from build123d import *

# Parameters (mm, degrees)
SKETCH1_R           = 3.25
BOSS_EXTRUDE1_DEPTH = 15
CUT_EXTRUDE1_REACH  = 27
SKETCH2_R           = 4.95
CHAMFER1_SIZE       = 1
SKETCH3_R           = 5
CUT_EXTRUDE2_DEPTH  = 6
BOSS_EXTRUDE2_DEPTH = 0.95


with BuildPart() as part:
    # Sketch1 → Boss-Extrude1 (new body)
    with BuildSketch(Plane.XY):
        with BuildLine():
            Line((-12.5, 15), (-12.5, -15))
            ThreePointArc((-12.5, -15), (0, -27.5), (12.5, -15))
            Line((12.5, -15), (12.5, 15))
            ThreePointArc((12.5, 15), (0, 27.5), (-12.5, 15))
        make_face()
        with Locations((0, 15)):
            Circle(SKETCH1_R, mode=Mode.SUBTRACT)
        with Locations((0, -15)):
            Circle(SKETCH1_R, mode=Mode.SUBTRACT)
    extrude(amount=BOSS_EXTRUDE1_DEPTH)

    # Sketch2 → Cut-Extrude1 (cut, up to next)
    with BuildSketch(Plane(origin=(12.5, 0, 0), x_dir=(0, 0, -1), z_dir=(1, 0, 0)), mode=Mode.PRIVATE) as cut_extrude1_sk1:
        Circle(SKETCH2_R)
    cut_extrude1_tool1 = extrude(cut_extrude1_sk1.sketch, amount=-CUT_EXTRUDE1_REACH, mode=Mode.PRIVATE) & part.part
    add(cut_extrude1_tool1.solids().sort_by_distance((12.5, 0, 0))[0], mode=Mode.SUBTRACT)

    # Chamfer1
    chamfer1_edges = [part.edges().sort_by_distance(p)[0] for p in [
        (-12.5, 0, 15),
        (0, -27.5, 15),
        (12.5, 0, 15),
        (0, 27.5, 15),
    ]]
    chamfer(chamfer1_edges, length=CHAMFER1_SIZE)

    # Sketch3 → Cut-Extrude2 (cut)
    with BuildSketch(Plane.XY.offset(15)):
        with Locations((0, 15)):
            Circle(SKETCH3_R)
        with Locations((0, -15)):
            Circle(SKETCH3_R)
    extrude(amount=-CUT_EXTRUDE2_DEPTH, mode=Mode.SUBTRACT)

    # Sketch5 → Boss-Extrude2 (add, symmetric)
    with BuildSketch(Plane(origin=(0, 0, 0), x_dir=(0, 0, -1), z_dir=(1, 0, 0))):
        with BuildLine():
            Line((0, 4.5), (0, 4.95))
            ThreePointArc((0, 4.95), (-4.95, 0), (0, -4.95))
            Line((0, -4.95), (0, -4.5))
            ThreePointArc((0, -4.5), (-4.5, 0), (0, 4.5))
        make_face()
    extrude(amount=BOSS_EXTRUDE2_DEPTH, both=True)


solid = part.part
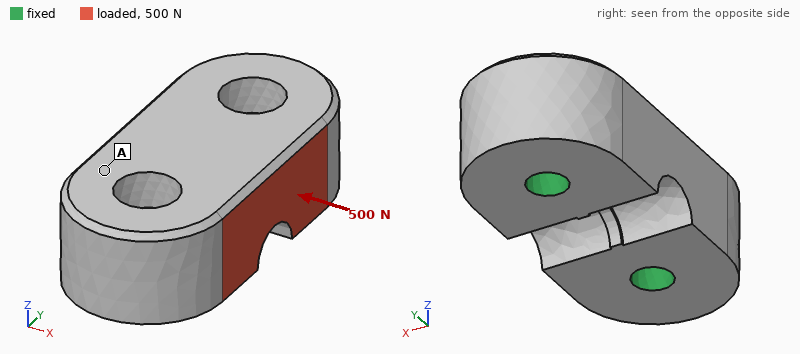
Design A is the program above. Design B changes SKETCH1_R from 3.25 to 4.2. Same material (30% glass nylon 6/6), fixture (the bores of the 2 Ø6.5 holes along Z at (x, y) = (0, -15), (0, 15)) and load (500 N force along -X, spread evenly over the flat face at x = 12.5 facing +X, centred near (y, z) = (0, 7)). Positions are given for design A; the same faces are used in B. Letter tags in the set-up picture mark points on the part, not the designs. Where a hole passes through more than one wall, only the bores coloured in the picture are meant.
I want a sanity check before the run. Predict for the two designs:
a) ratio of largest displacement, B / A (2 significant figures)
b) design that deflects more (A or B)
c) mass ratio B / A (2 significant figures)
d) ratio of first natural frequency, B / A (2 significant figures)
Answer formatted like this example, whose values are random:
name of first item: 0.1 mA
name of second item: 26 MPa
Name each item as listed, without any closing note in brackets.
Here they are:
ratio of largest displacement, B / A: 0.79
design that deflects more: A
mass ratio B / A: 0.98
ratio of first natural frequency, B / A: 1.2
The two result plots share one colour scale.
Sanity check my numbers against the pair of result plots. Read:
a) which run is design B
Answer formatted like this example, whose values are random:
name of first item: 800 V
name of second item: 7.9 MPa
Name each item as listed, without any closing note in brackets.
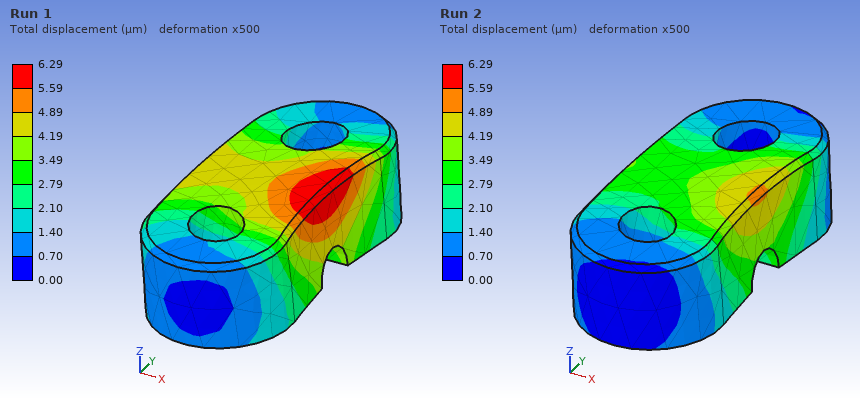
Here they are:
which run is design B: Run 2
